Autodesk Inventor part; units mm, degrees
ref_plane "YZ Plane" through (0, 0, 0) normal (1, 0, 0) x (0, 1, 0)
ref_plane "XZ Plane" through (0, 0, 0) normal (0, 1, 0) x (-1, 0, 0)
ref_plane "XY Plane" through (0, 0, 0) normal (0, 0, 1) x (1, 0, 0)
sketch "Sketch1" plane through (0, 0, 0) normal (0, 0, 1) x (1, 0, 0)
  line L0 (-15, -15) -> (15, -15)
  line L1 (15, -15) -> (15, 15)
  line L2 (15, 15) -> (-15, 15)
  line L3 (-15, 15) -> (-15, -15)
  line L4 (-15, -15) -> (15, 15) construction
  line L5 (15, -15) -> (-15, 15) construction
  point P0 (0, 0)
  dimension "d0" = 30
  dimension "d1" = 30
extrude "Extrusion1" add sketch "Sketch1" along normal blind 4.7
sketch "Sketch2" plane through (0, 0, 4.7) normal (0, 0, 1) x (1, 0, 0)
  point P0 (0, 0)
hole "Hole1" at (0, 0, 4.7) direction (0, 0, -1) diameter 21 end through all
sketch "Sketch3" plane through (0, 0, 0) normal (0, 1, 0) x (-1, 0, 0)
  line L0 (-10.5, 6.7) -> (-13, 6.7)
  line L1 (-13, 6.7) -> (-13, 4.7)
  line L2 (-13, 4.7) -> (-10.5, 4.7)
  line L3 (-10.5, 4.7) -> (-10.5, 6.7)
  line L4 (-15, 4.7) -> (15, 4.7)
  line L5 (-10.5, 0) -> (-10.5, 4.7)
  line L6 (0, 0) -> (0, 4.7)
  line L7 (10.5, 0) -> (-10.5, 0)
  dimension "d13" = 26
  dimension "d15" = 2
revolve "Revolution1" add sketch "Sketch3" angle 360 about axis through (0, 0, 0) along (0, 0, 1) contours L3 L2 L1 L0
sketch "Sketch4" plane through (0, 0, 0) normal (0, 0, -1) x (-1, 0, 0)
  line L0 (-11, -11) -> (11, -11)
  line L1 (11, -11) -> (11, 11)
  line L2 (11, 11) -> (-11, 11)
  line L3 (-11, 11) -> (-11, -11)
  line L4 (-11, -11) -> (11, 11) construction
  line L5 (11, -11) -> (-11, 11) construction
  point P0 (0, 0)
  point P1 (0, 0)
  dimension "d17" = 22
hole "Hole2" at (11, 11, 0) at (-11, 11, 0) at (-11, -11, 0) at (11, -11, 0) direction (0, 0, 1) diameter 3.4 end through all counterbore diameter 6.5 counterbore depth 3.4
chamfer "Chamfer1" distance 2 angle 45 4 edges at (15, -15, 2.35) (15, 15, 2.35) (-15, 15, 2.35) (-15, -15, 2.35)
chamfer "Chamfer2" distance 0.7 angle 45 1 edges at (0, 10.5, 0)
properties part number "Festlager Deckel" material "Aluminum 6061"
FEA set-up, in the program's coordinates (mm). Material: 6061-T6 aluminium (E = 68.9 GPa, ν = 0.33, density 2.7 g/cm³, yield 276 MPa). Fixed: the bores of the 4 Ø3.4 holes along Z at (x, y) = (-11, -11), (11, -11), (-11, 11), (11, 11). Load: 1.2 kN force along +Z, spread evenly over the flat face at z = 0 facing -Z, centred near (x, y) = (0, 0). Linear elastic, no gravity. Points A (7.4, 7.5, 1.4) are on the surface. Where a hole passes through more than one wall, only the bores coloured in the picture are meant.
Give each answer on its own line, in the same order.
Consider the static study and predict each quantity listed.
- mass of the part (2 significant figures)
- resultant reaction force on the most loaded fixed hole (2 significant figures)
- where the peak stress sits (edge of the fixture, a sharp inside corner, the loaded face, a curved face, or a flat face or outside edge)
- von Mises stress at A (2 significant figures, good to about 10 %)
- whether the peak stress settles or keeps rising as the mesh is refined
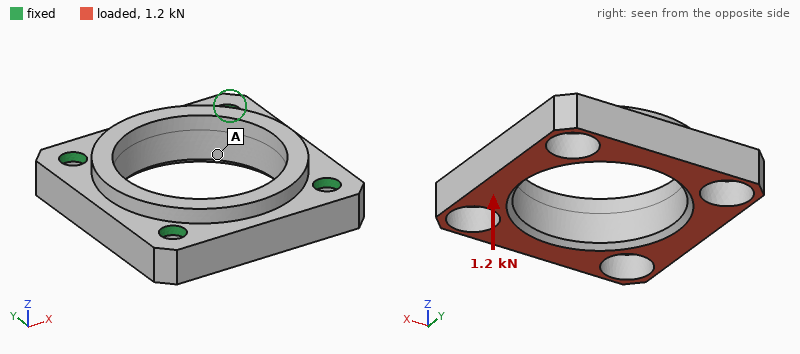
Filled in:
6.5 g
310 N
edge of the fixture
12 MPa
keeps rising
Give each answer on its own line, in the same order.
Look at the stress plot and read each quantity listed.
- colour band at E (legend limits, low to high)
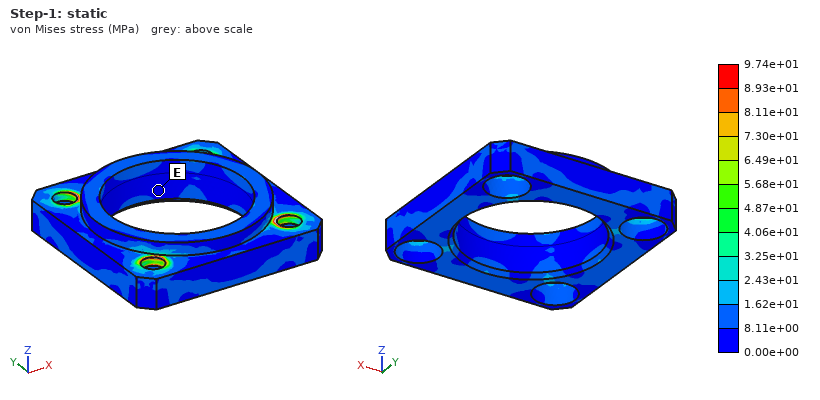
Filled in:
0.00e+00 to 8.11e+00 MPa
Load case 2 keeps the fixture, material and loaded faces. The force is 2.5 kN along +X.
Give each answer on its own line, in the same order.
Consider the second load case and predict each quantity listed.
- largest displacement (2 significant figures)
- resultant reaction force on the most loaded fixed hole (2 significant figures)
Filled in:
18 µm
660 N
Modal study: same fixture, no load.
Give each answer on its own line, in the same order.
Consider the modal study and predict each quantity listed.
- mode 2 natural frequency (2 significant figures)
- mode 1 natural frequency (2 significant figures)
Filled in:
31 kHz
25 kHz
